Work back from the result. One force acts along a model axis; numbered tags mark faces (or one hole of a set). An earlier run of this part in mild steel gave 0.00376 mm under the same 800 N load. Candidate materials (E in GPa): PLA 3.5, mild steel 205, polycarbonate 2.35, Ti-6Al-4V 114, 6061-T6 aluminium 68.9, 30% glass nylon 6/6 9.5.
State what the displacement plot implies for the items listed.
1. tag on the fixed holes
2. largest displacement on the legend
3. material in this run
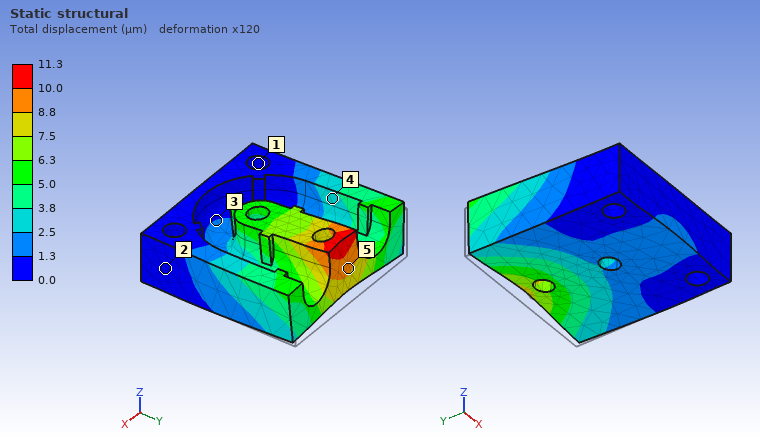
1
11.3 µm
6061-T6 aluminium
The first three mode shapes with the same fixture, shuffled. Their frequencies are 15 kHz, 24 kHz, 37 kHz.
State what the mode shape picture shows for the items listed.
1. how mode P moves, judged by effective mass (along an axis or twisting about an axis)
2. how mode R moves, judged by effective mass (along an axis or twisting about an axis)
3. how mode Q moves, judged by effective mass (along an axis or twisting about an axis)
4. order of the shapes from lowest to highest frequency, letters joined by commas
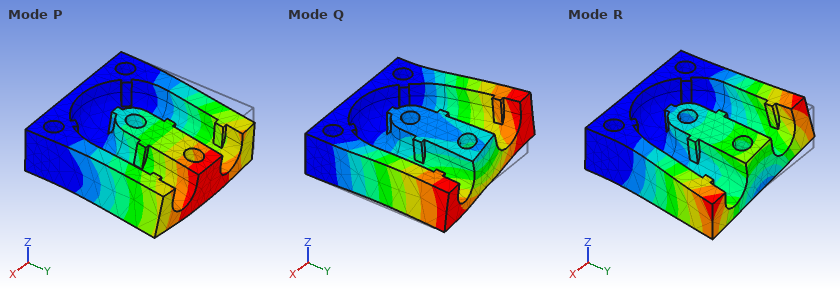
along Z
along X
along X
P, R, Q
